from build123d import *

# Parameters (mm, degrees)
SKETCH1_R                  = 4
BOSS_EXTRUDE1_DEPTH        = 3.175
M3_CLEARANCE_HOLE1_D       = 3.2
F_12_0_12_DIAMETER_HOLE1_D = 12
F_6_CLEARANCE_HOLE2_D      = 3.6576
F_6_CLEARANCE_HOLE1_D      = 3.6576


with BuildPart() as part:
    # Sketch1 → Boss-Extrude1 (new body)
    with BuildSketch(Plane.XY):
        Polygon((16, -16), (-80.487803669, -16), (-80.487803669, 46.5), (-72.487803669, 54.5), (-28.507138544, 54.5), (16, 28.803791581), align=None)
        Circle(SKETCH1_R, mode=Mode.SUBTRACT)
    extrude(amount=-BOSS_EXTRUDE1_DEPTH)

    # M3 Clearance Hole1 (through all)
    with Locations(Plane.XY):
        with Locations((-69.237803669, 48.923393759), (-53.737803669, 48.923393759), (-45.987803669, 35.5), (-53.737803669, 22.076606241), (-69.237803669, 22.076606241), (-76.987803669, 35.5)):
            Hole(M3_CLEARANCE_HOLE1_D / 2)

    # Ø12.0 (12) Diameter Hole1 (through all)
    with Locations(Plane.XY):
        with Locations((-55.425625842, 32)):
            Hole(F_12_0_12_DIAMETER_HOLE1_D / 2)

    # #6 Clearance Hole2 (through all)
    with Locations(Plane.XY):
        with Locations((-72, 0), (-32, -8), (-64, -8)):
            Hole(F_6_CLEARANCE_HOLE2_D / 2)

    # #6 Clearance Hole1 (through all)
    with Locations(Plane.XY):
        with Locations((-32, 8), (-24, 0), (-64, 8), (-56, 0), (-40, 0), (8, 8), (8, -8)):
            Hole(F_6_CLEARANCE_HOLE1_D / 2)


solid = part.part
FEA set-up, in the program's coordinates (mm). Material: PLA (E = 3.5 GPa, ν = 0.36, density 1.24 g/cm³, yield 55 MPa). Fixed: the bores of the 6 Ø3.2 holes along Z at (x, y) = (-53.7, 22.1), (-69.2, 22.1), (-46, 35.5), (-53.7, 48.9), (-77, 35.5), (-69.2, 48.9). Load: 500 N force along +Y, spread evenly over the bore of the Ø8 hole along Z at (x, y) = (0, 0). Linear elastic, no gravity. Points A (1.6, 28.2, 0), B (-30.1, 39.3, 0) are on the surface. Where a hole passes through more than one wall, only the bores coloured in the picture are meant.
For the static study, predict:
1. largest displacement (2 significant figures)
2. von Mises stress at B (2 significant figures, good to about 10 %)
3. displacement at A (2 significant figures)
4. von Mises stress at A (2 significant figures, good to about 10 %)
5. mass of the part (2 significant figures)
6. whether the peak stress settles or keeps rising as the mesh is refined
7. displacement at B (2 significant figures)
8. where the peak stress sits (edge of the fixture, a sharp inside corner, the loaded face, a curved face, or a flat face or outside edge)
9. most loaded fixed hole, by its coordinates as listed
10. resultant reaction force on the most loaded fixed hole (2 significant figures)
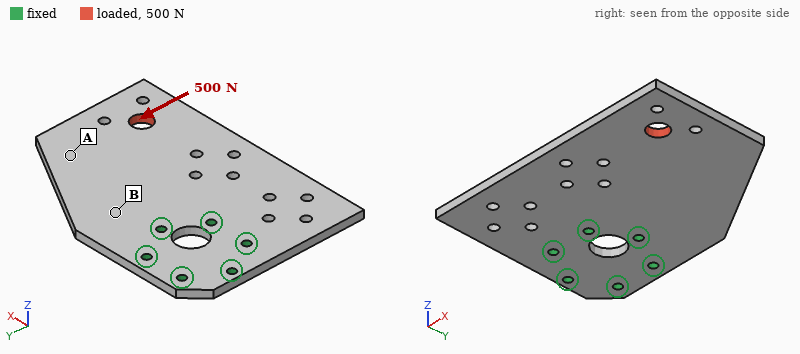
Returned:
0.54 mm
7.4 MPa
0.36 mm
3.3 MPa
23 g
keeps rising
0.13 mm
edge of the fixture
(-46, 35.5)
550 N
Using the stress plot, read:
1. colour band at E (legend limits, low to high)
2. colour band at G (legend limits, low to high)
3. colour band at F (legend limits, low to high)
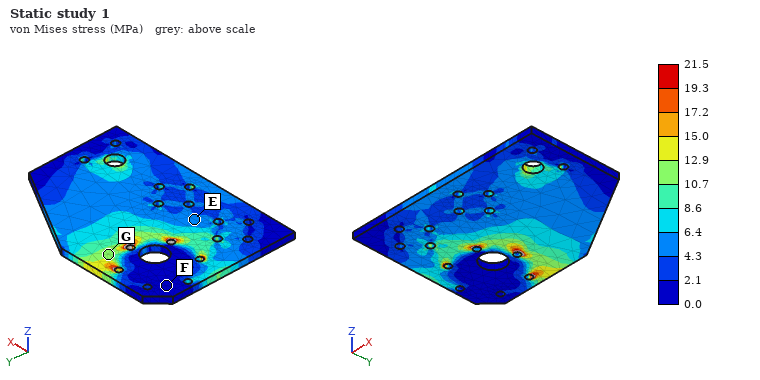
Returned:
4.3 to 6.4 MPa
10.7 to 12.9 MPa
0.0 to 2.1 MPa
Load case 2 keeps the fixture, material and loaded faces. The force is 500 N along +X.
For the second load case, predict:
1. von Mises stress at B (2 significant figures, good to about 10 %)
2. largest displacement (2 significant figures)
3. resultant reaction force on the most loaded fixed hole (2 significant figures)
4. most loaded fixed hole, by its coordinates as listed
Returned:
2.0 MPa
0.31 mm
420 N
(-53.7, 22.1)
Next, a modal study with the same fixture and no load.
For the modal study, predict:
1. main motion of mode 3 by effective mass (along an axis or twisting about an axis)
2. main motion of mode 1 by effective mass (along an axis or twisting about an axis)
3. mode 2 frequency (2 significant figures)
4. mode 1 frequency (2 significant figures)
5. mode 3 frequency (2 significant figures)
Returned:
along Z
along Z
480 Hz
200 Hz
750 Hz
